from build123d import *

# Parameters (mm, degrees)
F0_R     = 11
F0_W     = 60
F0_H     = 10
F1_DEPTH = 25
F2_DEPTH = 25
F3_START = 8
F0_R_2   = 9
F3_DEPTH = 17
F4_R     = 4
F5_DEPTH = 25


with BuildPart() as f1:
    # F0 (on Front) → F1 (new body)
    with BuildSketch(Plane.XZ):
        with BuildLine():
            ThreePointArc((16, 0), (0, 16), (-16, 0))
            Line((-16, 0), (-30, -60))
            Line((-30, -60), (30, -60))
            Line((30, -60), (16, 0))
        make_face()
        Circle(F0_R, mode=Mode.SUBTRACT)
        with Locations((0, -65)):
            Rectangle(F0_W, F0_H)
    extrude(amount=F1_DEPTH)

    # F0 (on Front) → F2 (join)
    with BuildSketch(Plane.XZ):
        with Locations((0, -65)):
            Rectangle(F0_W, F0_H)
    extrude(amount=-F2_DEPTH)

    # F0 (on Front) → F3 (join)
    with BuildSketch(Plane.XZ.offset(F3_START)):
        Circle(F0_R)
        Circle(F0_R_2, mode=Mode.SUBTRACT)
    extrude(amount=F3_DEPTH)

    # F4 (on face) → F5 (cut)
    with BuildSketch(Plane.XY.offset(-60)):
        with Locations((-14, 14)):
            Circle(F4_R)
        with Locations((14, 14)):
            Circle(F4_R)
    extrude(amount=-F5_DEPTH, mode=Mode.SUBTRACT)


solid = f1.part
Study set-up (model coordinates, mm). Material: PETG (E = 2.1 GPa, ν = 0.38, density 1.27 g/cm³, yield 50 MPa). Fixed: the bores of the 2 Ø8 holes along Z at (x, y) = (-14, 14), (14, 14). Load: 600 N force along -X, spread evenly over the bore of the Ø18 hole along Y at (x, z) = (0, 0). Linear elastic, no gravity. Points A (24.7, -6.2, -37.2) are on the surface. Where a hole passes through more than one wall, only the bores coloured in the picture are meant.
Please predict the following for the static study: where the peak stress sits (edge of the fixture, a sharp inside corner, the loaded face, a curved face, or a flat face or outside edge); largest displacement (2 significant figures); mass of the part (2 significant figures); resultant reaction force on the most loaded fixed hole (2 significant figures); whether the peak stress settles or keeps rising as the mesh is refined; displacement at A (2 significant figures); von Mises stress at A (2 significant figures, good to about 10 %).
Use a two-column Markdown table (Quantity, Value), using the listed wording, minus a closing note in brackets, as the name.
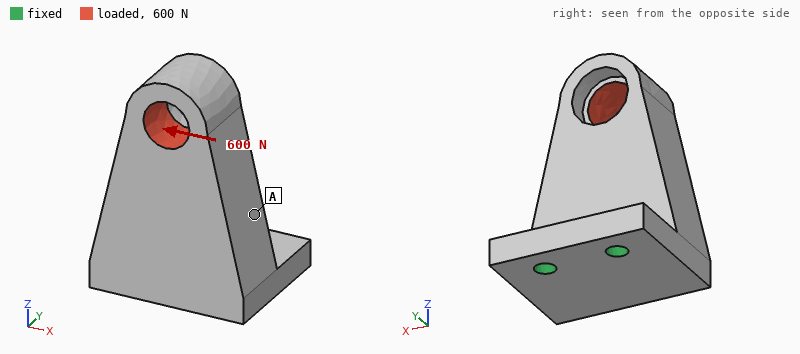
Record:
| Quantity | Value |
|---|---|
| where the peak stress sits | edge of the fixture |
| largest displacement | 1.3 mm |
| mass of the part | 130 g |
| resultant reaction force on the most loaded fixed hole | 1.2 kN |
| whether the peak stress settles or keeps rising as the mesh is refined | keeps rising |
| displacement at A | 0.55 mm |
| von Mises stress at A | 3.4 MPa |
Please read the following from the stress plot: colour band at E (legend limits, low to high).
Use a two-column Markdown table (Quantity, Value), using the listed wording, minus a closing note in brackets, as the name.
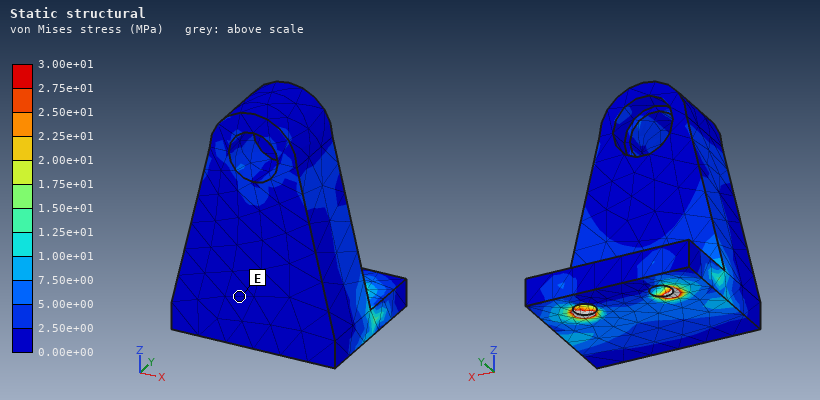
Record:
| Quantity | Value |
|---|---|
| colour band at E | 0.00e+00 to 2.50e+00 MPa |
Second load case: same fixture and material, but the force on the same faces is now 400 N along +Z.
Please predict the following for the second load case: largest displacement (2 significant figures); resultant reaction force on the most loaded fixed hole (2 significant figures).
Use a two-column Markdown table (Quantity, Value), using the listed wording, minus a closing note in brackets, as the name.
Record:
| Quantity | Value |
|---|---|
| largest displacement | 1.3 mm |
| resultant reaction force on the most loaded fixed hole | 200 N |
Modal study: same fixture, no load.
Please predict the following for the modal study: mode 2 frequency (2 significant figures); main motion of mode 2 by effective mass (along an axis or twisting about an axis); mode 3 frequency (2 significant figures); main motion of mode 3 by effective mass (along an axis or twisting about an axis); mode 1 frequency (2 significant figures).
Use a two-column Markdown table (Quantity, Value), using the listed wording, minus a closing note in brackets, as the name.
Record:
| Quantity | Value |
|---|---|
| mode 2 frequency | 620 Hz |
| main motion of mode 2 by effective mass | along X |
| mode 3 frequency | 1500 Hz |
| main motion of mode 3 by effective mass | along Z |
| mode 1 frequency | 290 Hz |
